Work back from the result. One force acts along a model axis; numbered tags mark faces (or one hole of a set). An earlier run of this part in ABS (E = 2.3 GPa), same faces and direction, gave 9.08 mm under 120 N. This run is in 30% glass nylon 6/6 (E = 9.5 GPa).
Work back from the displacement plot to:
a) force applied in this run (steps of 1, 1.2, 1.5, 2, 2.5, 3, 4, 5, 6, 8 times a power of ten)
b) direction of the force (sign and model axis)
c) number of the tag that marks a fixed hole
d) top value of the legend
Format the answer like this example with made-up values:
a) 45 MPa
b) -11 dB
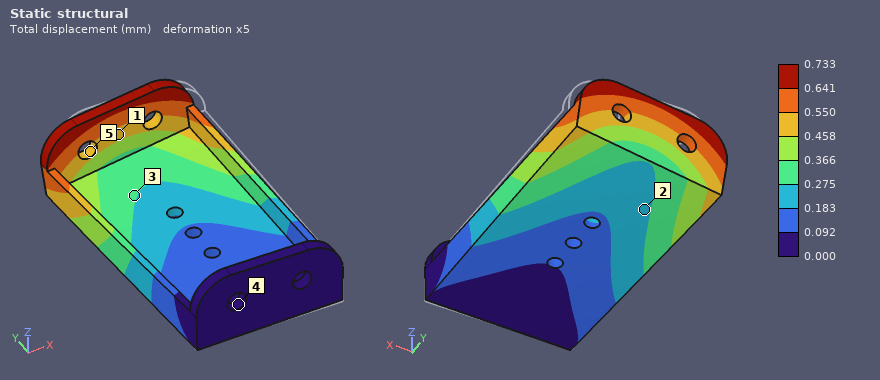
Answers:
a) 40 N
b) -X
c) 4
d) 0.733 mm
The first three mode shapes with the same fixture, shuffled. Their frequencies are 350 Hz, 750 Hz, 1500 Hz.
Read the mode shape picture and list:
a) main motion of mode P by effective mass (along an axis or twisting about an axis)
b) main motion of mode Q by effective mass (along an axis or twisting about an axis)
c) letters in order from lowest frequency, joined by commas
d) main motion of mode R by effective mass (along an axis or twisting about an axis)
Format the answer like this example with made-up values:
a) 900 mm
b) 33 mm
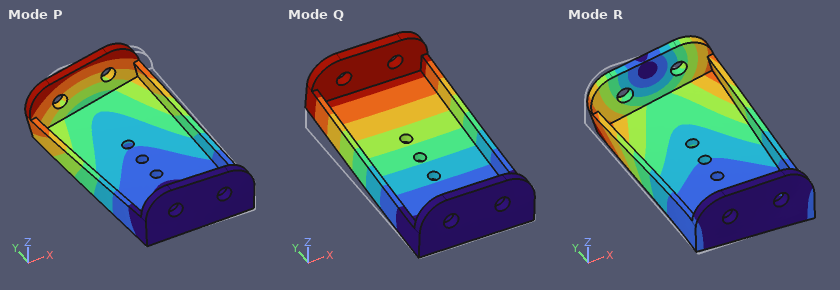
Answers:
a) along X
b) along Z
c) Q, P, R
d) along X
